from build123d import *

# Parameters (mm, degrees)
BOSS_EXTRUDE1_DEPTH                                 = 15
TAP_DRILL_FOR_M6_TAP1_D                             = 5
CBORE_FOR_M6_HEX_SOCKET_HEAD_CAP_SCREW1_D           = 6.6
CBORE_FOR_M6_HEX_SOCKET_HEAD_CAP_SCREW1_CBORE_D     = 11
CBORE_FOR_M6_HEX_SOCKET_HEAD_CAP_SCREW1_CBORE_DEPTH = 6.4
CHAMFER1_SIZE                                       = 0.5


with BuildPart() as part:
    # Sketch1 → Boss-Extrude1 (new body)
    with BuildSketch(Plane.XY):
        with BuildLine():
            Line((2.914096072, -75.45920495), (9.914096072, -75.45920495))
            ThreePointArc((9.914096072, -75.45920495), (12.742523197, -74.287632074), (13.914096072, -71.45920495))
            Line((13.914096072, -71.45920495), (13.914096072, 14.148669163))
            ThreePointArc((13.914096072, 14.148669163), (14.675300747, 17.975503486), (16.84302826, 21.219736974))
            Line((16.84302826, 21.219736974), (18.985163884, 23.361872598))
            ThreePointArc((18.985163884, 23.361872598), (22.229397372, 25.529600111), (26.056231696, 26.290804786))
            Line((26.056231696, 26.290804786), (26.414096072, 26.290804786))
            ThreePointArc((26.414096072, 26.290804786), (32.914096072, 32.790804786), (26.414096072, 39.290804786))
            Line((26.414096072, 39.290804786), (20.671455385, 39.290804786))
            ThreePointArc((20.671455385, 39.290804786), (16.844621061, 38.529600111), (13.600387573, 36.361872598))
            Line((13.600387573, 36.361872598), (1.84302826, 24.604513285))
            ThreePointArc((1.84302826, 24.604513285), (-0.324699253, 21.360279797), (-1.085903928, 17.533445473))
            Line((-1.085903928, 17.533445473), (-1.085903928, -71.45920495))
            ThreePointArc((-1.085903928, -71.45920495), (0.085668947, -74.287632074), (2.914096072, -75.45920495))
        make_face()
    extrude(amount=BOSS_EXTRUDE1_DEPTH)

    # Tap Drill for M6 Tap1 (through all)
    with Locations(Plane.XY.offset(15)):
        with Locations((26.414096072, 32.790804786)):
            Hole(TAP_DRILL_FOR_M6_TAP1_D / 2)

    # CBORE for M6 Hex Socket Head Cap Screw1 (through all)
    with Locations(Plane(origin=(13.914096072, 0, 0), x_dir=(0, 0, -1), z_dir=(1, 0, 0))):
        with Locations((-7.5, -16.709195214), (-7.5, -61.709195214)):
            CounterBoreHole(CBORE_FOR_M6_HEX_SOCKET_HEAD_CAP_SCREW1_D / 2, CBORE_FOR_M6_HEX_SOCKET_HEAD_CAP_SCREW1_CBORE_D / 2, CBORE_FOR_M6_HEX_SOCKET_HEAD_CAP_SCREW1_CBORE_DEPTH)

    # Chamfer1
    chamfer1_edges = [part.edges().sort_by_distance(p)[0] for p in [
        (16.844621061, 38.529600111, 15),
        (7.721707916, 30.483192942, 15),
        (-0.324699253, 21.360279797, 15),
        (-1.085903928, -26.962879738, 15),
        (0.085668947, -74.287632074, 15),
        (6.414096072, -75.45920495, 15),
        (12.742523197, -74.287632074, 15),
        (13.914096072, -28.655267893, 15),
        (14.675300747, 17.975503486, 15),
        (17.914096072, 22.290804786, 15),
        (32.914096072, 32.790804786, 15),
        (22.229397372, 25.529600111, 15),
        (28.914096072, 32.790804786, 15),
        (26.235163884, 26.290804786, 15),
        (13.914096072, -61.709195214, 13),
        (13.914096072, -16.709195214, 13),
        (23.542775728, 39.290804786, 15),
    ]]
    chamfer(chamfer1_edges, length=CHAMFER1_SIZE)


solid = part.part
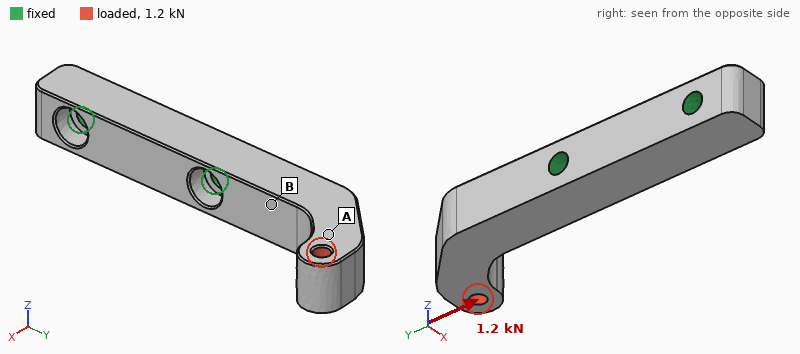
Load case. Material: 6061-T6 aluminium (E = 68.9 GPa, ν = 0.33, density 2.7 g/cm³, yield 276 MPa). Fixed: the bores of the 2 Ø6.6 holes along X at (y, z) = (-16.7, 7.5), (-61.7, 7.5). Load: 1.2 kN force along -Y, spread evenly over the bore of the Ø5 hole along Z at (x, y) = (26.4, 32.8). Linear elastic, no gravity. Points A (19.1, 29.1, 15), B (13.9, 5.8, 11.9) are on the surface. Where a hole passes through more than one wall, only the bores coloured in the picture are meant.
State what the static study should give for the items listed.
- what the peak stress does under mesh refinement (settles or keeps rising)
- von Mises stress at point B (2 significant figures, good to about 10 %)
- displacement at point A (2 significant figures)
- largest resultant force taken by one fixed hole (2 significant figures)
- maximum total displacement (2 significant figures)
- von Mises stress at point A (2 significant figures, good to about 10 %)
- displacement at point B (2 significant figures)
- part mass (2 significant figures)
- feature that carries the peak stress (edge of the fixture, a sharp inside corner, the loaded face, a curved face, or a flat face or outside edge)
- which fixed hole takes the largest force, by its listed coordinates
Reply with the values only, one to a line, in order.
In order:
keeps rising
48 MPa
0.15 mm
750 N
0.22 mm
19 MPa
0.048 mm
68 g
edge of the fixture
(-16.7, 7.5)
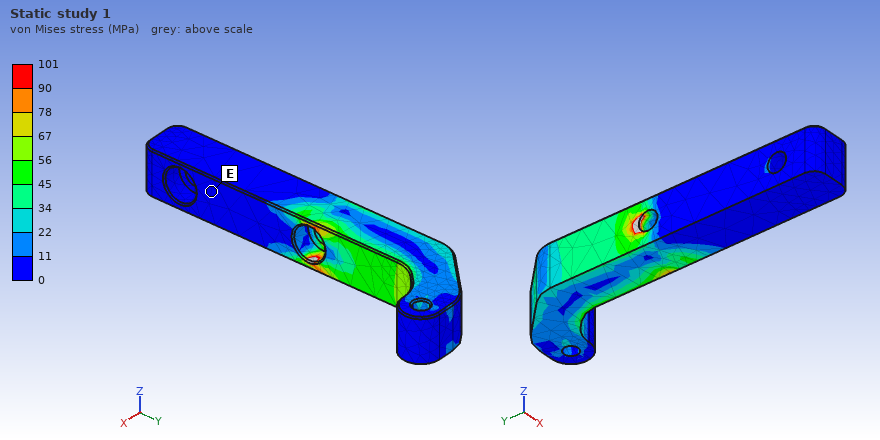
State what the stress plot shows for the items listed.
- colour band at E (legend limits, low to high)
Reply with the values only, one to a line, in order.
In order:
0 to 11 MPa
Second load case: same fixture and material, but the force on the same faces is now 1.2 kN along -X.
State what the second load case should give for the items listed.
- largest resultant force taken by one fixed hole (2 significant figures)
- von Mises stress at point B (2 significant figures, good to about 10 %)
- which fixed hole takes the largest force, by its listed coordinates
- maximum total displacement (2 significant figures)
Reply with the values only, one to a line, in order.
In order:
1.8 kN
58 MPa
(-16.7, 7.5)
0.35 mm
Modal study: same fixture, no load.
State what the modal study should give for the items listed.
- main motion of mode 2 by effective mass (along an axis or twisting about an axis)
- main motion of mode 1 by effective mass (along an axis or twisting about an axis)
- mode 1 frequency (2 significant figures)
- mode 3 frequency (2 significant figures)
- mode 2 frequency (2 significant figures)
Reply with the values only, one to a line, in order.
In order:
along Z
along X
2600 Hz
8100 Hz
2700 Hz
